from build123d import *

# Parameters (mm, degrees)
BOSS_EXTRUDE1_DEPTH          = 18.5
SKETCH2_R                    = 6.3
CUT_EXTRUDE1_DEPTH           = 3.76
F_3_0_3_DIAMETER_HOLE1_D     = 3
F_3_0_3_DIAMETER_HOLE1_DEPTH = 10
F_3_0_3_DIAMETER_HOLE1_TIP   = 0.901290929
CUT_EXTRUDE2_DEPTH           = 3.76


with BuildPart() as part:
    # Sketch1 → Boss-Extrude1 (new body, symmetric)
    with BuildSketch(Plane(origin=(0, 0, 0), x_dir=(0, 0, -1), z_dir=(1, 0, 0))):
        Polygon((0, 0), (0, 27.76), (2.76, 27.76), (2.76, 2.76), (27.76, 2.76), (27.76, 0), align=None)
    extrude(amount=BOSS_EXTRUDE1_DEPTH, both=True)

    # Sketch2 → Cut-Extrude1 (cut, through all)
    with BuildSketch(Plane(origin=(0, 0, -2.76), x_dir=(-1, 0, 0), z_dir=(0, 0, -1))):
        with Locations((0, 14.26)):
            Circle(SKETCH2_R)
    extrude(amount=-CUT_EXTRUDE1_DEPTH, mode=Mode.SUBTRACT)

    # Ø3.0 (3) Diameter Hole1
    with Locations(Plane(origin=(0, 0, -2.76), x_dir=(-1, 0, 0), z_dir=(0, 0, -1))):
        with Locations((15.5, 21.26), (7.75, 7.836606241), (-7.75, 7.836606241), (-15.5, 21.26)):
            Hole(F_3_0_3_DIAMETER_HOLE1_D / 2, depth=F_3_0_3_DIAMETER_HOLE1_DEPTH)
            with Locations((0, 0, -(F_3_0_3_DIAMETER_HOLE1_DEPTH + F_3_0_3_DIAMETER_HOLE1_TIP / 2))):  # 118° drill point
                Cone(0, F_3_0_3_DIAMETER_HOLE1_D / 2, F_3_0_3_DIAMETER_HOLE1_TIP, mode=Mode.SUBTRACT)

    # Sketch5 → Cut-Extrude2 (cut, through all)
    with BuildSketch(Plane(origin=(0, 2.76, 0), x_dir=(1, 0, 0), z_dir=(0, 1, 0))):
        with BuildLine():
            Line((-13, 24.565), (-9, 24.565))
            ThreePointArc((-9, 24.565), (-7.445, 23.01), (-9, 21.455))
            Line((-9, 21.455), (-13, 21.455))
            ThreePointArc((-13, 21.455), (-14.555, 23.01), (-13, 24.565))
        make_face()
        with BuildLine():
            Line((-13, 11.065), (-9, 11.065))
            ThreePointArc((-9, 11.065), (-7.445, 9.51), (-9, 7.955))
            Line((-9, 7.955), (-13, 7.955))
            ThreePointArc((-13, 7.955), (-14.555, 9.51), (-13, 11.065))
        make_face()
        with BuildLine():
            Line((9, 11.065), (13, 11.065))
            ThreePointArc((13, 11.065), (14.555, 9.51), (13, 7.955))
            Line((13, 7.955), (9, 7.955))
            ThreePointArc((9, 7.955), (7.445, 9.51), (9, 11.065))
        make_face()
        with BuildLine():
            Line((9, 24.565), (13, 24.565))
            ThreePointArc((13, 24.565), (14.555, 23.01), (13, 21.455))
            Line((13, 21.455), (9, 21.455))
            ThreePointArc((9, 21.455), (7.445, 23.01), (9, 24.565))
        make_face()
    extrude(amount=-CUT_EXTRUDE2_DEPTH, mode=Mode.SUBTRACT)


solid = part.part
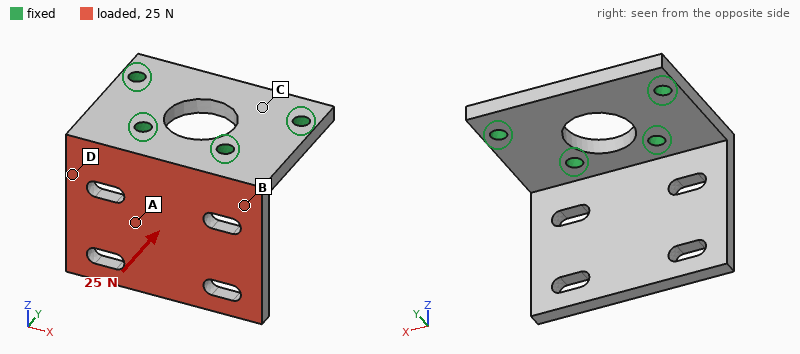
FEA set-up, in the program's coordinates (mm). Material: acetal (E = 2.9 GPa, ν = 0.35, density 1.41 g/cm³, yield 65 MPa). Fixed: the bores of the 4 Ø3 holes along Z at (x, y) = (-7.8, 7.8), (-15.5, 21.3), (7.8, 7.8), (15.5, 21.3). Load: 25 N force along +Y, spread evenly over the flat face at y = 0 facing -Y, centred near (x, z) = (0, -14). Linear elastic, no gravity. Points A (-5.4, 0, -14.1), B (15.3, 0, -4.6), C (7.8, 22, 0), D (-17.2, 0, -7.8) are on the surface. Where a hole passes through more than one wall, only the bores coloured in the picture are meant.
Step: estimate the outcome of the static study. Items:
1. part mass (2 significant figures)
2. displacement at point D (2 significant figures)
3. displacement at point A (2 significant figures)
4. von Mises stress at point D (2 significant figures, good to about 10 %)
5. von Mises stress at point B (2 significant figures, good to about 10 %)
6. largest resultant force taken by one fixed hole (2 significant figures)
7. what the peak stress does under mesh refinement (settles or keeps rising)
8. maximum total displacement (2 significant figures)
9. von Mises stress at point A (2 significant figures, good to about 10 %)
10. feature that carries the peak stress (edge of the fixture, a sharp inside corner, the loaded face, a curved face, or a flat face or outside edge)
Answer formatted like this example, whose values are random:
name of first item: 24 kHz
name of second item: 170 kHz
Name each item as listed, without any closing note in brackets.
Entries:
part mass: 6.7 g
displacement at point D: 0.10 mm
displacement at point A: 0.24 mm
von Mises stress at point D: 5.4 MPa
von Mises stress at point B: 4.6 MPa
largest resultant force taken by one fixed hole: 12 N
what the peak stress does under mesh refinement: keeps rising
maximum total displacement: 0.58 mm
von Mises stress at point A: 1.9 MPa
feature that carries the peak stress: edge of the fixture
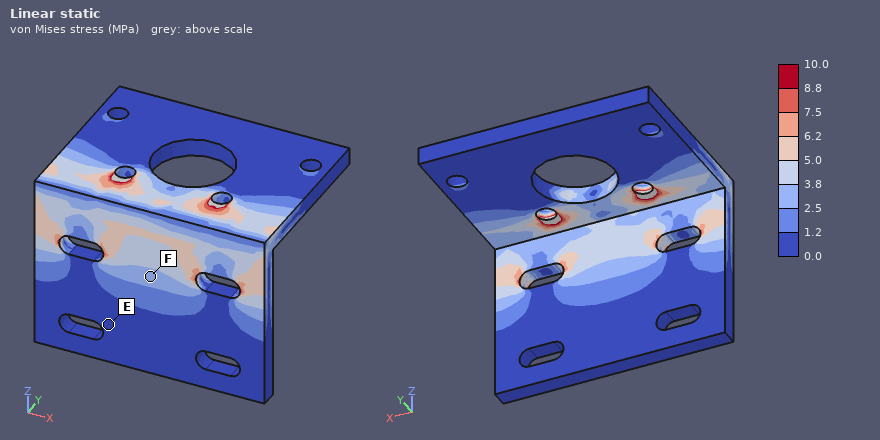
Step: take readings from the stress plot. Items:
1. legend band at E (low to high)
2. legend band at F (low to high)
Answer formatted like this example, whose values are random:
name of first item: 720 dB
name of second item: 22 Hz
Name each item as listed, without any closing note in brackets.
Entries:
legend band at E: 0.0 to 1.2 MPa
legend band at F: 2.5 to 3.8 MPa
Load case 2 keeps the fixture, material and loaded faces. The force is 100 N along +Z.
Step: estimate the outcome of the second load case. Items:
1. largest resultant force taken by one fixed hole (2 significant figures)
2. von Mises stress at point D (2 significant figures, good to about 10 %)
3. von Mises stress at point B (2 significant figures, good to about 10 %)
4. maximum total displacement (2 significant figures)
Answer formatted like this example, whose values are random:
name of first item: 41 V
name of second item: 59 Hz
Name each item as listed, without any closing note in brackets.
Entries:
largest resultant force taken by one fixed hole: 56 N
von Mises stress at point D: 3.6 MPa
von Mises stress at point B: 3.3 MPa
maximum total displacement: 0.64 mm
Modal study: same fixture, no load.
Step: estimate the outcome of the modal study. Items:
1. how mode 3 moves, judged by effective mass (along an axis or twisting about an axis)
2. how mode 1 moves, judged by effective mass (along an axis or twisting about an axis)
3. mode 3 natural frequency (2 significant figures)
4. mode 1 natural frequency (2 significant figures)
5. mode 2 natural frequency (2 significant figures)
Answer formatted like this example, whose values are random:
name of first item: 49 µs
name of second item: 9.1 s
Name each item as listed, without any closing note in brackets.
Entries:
how mode 3 moves, judged by effective mass: along X
how mode 1 moves, judged by effective mass: along Y
mode 3 natural frequency: 2100 Hz
mode 1 natural frequency: 680 Hz
mode 2 natural frequency: 1400 Hz
